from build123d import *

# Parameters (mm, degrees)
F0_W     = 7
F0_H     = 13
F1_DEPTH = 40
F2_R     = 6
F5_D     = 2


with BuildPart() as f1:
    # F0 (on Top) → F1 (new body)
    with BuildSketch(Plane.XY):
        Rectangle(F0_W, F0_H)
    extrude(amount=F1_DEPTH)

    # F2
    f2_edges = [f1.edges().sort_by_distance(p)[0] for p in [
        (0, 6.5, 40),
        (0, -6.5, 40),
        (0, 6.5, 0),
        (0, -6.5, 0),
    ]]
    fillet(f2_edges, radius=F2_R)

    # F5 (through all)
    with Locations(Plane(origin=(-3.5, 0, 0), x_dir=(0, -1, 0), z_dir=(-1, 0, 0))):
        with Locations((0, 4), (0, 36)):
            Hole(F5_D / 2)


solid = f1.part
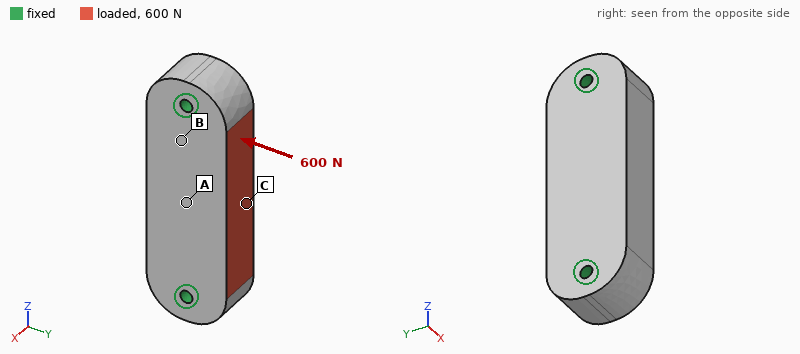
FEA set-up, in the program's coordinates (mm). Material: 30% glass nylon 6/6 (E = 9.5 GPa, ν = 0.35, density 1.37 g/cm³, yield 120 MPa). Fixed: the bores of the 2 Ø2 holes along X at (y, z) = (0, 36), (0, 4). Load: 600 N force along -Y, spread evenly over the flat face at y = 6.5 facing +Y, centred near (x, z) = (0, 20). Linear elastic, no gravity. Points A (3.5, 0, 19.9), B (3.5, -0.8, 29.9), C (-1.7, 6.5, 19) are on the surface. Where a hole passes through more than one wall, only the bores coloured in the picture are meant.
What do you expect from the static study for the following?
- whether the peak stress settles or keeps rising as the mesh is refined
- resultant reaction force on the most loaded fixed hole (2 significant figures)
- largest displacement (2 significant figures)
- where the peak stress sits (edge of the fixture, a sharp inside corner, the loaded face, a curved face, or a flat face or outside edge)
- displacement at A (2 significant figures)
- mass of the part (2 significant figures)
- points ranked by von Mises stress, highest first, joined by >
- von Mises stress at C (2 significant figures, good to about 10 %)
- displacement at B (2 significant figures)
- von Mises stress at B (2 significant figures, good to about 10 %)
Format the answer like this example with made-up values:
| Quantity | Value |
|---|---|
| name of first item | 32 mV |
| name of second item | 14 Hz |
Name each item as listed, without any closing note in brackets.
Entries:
| Quantity | Value |
|---|---|
| whether the peak stress settles or keeps rising as the mesh is refined | keeps rising |
| resultant reaction force on the most loaded fixed hole | 300 N |
| largest displacement | 27 µm |
| where the peak stress sits | edge of the fixture |
| displacement at A | 27 µm |
| mass of the part | 4.6 g |
| points ranked by von Mises stress, highest first, joined by > | C > B > A |
| von Mises stress at C | 11 MPa |
| displacement at B | 15 µm |
| von Mises stress at B | 6.1 MPa |
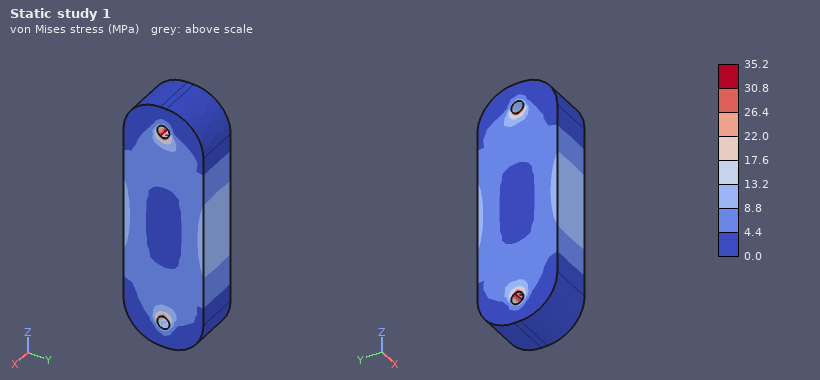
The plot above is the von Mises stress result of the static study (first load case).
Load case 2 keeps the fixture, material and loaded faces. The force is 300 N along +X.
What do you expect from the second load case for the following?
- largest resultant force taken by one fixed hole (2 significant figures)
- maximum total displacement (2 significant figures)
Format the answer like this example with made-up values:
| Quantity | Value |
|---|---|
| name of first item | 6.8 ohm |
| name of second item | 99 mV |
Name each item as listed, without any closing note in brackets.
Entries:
| Quantity | Value |
|---|---|
| largest resultant force taken by one fixed hole | 150 N |
| maximum total displacement | 42 µm |
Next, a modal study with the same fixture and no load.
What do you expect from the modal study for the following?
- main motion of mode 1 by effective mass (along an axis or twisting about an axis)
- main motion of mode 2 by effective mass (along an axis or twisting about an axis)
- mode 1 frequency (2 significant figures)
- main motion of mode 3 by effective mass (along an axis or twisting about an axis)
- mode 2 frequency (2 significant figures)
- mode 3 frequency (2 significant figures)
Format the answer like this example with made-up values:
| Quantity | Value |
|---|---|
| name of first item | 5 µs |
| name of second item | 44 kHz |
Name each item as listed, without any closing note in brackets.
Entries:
| Quantity | Value |
|---|---|
| main motion of mode 1 by effective mass | along X |
| main motion of mode 2 by effective mass | along Y |
| mode 1 frequency | 12 kHz |
| main motion of mode 3 by effective mass | twisting about Z |
| mode 2 frequency | 14 kHz |
| mode 3 frequency | 17 kHz |
